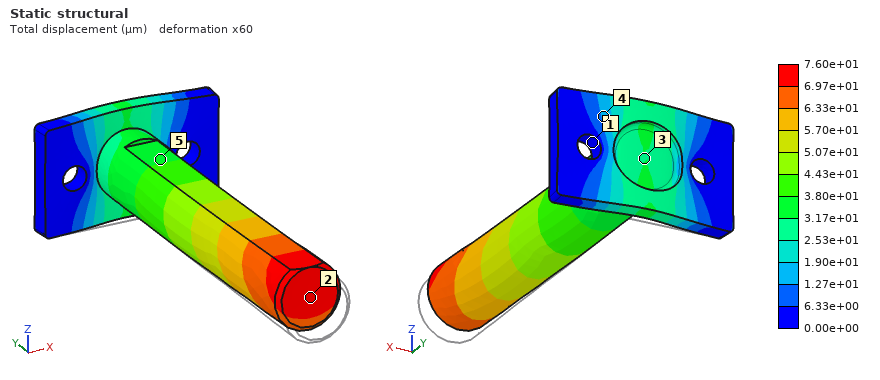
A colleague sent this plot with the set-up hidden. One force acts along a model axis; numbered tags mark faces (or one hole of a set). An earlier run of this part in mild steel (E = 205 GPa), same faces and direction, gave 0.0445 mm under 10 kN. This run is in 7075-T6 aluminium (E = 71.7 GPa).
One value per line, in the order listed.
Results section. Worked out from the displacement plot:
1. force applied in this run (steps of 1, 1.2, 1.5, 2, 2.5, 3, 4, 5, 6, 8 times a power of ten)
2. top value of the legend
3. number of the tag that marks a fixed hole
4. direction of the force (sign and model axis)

6 kN
7.60e+01 µm
1
+Y
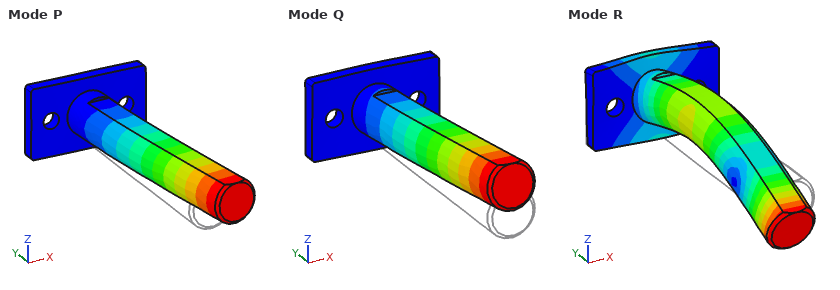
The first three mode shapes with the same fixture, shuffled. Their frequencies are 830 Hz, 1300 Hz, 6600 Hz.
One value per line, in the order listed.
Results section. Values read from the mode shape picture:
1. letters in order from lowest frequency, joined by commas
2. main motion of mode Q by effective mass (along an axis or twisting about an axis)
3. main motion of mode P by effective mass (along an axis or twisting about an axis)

Q, P, R
along Z
along X
